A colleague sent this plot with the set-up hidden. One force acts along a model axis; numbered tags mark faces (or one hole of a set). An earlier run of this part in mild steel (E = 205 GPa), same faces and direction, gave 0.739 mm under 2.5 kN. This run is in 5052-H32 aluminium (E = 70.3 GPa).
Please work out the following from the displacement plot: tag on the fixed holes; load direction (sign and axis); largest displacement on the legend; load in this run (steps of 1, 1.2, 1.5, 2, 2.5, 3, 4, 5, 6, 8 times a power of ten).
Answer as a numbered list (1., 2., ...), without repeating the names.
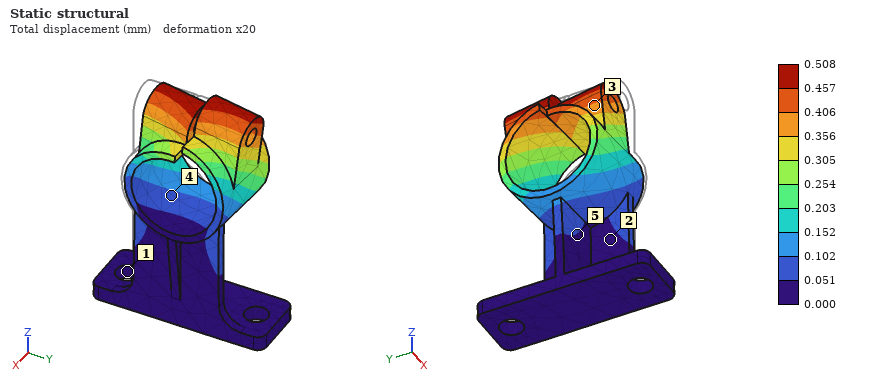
1. 1
2. +Y
3. 0.508 mm
4. 600 N
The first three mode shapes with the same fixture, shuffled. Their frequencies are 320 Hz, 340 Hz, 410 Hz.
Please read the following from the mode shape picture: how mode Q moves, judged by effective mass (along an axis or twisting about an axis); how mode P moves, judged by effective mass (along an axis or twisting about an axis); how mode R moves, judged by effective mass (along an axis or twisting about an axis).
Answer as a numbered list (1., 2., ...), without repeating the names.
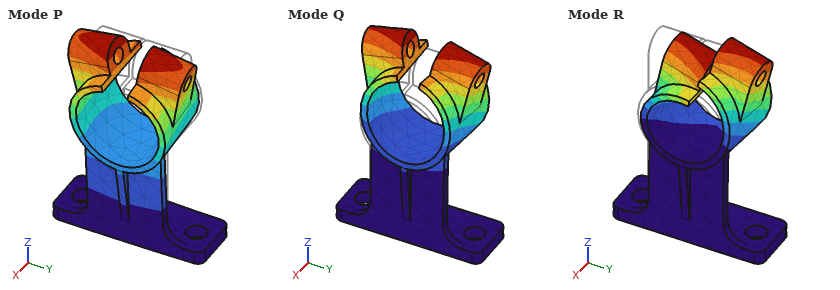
1. along X
2. along X
3. along Y
